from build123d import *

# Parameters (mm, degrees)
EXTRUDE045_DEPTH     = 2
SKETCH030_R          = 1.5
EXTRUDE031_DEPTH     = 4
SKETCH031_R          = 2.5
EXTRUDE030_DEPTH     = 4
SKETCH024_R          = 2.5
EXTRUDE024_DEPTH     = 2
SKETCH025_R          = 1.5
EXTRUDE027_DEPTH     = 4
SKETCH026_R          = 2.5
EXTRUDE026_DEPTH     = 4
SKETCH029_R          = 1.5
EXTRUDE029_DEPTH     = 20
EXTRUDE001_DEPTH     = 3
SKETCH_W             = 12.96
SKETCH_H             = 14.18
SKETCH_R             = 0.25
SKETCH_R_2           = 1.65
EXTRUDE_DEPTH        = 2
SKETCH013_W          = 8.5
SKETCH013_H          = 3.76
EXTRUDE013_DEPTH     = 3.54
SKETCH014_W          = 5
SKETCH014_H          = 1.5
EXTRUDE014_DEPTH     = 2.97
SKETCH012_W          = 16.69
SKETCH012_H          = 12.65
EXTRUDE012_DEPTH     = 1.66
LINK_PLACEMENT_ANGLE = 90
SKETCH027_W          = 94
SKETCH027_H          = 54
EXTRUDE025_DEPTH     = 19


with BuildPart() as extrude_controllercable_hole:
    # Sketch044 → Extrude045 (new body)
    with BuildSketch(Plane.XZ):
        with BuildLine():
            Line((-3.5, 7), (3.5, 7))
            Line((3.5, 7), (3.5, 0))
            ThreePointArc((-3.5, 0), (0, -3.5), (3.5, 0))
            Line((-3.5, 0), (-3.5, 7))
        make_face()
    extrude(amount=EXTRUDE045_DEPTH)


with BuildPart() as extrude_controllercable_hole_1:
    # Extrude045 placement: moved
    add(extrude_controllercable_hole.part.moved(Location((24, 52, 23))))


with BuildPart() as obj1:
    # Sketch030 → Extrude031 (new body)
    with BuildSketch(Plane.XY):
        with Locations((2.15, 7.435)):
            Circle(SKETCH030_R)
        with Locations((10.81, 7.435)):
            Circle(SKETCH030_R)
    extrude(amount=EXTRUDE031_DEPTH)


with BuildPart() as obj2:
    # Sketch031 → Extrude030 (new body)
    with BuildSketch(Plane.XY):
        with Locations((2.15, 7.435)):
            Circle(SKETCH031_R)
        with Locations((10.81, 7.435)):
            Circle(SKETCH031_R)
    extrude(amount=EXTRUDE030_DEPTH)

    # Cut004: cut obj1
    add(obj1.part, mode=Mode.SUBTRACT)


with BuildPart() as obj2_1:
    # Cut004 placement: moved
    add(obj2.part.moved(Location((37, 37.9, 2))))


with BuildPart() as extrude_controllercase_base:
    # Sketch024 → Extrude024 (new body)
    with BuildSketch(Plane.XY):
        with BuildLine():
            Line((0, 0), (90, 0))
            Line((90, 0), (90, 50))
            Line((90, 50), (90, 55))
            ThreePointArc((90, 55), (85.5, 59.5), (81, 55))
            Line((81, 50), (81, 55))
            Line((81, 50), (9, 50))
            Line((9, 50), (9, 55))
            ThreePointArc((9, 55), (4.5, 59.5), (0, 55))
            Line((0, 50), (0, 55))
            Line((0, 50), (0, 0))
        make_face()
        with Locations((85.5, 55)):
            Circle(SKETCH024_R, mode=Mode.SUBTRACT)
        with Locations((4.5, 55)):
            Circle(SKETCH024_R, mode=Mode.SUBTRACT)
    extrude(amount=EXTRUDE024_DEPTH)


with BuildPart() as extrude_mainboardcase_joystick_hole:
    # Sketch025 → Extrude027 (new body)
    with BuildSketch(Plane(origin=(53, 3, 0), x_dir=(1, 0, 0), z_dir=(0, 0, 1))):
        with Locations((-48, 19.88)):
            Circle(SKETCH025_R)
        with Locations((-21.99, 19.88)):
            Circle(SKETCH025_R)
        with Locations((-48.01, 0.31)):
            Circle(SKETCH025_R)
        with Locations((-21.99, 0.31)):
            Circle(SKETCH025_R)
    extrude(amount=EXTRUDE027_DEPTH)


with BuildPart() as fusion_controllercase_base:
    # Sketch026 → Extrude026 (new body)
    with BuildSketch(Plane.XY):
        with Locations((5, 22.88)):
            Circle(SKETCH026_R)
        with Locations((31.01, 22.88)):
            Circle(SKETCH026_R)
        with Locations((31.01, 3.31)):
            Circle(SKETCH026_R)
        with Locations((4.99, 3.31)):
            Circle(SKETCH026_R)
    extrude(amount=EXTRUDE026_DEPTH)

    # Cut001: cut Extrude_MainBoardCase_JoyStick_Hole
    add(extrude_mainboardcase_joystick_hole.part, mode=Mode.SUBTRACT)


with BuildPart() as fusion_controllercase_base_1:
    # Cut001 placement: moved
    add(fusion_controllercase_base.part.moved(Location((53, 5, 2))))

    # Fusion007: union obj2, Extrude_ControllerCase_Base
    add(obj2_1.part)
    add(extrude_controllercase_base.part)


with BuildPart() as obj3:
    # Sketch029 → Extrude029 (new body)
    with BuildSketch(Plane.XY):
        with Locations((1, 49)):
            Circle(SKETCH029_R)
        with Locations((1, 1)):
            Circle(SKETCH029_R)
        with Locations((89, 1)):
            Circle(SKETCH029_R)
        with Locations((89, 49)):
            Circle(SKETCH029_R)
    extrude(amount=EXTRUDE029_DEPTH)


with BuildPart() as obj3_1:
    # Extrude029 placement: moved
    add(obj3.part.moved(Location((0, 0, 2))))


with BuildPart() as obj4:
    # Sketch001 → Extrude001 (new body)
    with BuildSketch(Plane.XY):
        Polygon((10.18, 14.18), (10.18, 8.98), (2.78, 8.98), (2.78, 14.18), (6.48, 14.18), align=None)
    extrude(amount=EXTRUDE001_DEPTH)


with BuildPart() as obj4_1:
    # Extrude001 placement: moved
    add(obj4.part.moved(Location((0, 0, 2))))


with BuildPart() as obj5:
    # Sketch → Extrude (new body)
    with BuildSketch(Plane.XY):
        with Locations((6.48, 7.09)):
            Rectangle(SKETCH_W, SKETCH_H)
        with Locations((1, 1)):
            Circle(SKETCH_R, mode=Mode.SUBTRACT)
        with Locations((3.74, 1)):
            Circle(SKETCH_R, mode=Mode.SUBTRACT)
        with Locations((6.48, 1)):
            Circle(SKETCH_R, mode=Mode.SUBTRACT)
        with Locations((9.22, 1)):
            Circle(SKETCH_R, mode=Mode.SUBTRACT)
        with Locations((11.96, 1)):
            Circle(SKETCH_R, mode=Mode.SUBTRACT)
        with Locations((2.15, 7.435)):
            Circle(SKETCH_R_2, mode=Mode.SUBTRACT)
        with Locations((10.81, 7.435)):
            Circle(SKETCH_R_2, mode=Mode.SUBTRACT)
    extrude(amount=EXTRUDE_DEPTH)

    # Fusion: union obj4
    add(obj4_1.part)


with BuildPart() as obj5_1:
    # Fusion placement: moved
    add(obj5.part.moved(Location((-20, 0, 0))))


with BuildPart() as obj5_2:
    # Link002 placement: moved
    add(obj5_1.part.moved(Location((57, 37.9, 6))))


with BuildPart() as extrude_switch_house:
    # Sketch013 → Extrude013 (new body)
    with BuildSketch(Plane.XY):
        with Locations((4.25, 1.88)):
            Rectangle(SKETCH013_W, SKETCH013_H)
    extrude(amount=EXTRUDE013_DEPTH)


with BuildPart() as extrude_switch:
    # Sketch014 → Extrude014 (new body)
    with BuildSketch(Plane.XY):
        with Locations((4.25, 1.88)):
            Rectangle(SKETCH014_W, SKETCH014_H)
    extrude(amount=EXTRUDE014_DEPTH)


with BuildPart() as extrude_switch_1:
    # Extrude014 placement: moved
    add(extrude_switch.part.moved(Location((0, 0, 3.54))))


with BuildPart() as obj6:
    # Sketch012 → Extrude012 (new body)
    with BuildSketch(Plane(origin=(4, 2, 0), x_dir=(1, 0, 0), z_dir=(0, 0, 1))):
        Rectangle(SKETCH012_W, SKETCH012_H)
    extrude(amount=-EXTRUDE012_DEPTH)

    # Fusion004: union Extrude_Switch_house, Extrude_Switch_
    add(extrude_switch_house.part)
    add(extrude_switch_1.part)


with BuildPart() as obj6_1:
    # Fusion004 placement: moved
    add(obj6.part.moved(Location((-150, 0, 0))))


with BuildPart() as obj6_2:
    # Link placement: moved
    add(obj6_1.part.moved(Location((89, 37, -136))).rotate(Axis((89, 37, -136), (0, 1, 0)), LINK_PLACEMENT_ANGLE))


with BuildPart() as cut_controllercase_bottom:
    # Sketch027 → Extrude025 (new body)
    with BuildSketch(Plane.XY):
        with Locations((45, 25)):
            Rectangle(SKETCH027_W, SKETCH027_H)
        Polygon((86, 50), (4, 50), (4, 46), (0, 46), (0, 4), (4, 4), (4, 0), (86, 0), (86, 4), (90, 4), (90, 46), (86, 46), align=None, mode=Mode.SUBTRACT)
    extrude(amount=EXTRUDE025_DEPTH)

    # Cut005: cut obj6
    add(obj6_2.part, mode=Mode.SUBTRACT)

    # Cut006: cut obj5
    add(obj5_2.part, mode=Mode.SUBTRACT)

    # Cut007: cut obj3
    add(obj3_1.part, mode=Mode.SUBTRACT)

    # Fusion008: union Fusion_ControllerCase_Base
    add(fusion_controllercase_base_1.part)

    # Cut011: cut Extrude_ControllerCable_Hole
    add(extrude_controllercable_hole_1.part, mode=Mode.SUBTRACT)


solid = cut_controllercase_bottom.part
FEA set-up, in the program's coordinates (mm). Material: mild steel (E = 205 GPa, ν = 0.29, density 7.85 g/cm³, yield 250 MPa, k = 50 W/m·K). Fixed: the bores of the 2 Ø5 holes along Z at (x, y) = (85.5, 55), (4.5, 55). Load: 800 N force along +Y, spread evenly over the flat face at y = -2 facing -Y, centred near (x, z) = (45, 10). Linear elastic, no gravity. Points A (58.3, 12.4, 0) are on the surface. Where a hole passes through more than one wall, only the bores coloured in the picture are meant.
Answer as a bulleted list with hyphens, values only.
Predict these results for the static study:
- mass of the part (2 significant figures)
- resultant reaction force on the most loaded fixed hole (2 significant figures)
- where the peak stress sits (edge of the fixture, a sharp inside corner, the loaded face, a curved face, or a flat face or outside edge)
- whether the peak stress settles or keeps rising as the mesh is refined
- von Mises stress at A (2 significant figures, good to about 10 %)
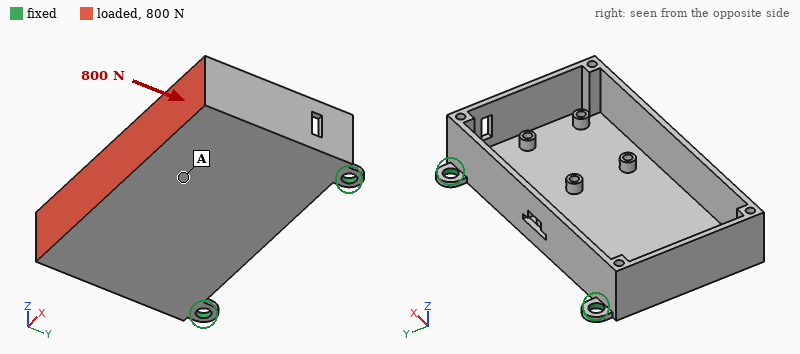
- 160 g
- 410 N
- edge of the fixture
- keeps rising
- 26 MPa
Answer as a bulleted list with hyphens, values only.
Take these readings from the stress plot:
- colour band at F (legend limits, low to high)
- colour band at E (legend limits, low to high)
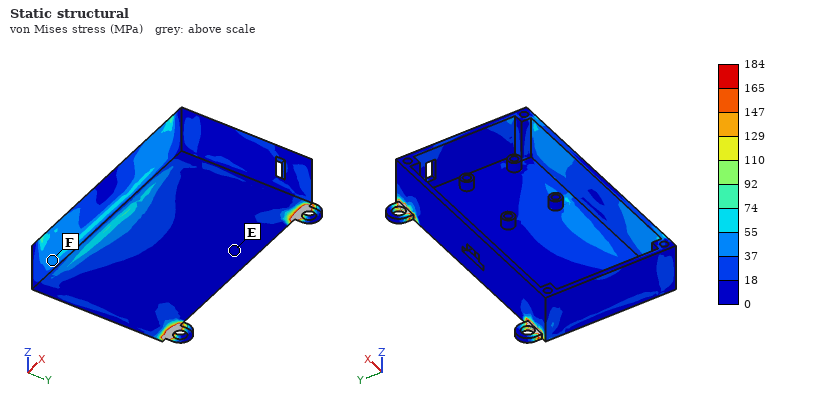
- 37 to 55 MPa
- 0 to 18 MPa
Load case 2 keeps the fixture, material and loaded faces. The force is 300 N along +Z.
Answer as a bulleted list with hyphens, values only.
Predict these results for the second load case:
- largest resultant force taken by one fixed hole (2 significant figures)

- 160 N
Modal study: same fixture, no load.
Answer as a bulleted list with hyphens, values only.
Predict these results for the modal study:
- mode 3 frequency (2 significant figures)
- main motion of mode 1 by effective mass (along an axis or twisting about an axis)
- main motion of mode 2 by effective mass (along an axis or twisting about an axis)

- 2700 Hz
- along Z
- twisting about Y
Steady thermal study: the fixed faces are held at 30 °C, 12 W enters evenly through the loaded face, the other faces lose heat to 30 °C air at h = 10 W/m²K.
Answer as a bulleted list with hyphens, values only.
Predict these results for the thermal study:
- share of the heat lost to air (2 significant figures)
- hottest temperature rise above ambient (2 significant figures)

- 49 %
- 60 K
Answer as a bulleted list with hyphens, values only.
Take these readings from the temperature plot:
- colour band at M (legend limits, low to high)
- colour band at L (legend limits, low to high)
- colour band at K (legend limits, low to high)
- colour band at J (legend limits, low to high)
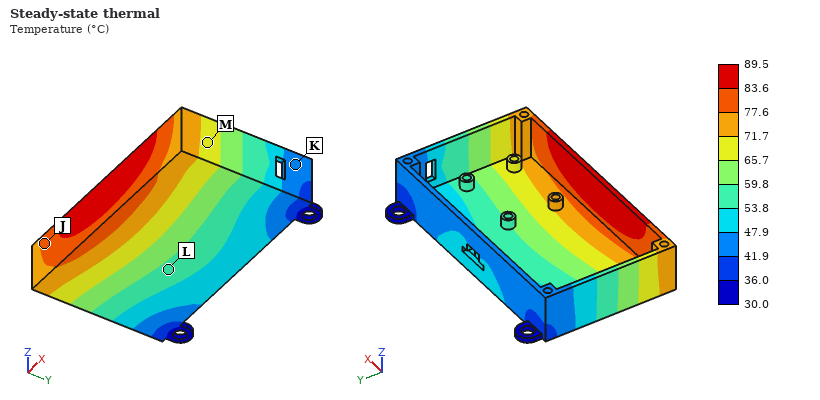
- 65.7 to 71.7 °C
- 53.8 to 59.8 °C
- 41.9 to 47.9 °C
- 77.6 to 83.6 °C
